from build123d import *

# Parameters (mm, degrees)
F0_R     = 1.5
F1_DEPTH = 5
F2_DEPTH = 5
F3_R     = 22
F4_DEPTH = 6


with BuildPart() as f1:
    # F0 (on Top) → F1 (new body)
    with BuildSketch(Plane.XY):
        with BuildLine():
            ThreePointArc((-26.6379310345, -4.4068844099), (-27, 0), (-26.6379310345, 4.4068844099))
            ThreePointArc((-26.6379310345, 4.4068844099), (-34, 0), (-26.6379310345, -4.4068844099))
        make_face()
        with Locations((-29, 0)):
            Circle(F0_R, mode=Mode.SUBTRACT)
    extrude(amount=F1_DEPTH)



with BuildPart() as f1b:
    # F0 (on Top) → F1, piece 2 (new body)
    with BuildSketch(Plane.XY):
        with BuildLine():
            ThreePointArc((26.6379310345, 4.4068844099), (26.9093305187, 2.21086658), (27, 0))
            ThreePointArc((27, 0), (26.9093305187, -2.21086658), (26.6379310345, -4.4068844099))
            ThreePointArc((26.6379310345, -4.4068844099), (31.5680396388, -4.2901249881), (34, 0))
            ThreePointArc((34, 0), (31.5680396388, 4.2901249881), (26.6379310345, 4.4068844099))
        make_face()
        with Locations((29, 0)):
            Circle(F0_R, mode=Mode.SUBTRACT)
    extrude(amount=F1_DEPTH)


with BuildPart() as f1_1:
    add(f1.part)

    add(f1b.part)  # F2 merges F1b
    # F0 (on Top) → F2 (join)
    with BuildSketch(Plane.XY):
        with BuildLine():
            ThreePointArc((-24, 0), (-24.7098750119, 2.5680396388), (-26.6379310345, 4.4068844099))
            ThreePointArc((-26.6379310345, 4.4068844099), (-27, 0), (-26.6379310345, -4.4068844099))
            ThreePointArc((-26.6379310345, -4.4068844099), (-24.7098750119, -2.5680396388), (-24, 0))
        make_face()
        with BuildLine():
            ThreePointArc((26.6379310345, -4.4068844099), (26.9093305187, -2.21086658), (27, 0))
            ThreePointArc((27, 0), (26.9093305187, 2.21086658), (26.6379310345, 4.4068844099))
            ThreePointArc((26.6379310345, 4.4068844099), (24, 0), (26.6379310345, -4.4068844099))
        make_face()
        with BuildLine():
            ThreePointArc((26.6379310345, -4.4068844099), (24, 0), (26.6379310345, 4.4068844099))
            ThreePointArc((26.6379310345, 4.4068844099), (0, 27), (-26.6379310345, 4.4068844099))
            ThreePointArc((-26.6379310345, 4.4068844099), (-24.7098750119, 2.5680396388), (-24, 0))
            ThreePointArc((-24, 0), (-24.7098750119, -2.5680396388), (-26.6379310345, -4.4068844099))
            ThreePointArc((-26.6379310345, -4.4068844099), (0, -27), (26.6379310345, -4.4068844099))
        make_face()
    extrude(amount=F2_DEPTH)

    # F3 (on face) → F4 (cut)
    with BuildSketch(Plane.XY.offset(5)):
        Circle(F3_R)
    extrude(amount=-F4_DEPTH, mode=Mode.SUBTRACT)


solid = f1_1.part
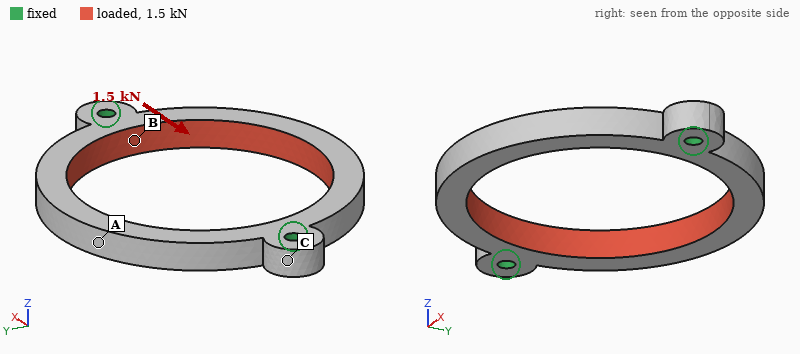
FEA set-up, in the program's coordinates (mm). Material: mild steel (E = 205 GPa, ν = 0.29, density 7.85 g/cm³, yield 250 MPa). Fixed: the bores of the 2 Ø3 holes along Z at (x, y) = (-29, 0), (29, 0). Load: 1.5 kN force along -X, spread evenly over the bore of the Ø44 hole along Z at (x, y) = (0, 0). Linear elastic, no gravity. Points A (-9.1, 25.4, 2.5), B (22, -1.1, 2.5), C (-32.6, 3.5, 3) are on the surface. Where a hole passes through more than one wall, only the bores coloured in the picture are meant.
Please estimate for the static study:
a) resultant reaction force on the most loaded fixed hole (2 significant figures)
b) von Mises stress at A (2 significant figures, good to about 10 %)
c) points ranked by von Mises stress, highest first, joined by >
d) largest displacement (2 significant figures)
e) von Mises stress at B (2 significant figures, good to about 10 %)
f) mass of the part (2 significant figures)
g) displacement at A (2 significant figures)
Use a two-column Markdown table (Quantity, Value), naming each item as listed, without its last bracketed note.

| Quantity | Value |
|---|---|
| resultant reaction force on the most loaded fixed hole | 750 N |
| von Mises stress at A | 32 MPa |
| points ranked by von Mises stress, highest first, joined by > | B > A > C |
| largest displacement | 16 µm |
| von Mises stress at B | 70 MPa |
| mass of the part | 34 g |
| displacement at A | 14 µm |
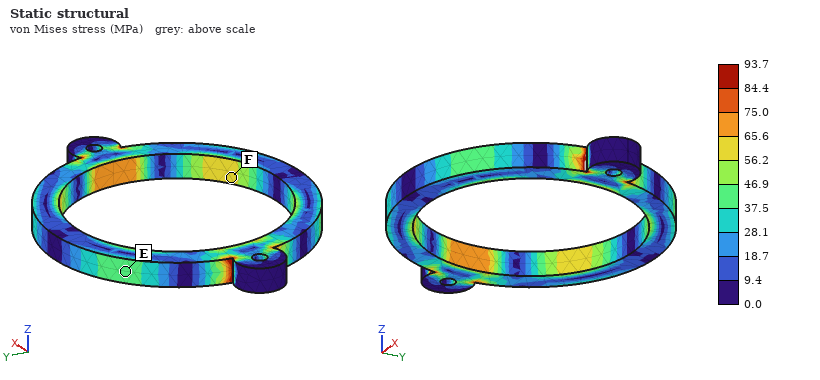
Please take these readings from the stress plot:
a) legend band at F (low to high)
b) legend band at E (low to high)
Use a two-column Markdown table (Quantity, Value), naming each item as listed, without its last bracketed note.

| Quantity | Value |
|---|---|
| legend band at F | 56.2 to 65.6 MPa |
| legend band at E | 37.5 to 46.9 MPa |
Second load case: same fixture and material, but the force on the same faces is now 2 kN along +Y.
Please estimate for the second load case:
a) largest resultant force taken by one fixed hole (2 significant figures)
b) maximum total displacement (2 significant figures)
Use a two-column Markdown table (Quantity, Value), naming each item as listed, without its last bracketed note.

| Quantity | Value |
|---|---|
| largest resultant force taken by one fixed hole | 1.0 kN |
| maximum total displacement | 5.4 µm |
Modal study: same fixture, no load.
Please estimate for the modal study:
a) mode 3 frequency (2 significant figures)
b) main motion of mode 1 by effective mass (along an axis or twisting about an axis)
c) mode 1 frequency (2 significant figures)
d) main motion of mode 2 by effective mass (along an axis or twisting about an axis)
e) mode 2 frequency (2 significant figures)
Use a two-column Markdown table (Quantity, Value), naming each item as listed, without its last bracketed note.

| Quantity | Value |
|---|---|
| mode 3 frequency | 8000 Hz |
| main motion of mode 1 by effective mass | twisting about X |
| mode 1 frequency | 3200 Hz |
| main motion of mode 2 by effective mass | along Z |
| mode 2 frequency | 3600 Hz |
